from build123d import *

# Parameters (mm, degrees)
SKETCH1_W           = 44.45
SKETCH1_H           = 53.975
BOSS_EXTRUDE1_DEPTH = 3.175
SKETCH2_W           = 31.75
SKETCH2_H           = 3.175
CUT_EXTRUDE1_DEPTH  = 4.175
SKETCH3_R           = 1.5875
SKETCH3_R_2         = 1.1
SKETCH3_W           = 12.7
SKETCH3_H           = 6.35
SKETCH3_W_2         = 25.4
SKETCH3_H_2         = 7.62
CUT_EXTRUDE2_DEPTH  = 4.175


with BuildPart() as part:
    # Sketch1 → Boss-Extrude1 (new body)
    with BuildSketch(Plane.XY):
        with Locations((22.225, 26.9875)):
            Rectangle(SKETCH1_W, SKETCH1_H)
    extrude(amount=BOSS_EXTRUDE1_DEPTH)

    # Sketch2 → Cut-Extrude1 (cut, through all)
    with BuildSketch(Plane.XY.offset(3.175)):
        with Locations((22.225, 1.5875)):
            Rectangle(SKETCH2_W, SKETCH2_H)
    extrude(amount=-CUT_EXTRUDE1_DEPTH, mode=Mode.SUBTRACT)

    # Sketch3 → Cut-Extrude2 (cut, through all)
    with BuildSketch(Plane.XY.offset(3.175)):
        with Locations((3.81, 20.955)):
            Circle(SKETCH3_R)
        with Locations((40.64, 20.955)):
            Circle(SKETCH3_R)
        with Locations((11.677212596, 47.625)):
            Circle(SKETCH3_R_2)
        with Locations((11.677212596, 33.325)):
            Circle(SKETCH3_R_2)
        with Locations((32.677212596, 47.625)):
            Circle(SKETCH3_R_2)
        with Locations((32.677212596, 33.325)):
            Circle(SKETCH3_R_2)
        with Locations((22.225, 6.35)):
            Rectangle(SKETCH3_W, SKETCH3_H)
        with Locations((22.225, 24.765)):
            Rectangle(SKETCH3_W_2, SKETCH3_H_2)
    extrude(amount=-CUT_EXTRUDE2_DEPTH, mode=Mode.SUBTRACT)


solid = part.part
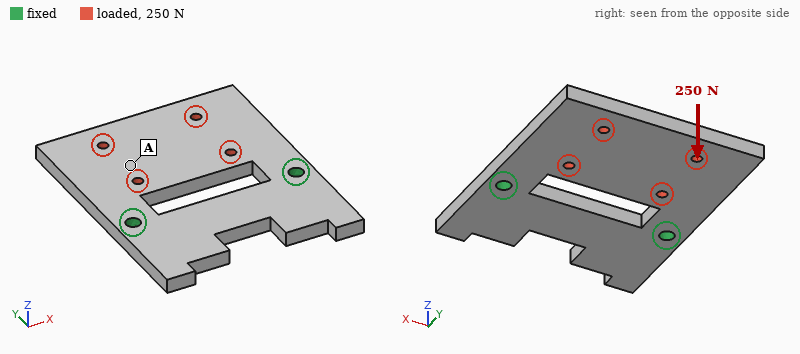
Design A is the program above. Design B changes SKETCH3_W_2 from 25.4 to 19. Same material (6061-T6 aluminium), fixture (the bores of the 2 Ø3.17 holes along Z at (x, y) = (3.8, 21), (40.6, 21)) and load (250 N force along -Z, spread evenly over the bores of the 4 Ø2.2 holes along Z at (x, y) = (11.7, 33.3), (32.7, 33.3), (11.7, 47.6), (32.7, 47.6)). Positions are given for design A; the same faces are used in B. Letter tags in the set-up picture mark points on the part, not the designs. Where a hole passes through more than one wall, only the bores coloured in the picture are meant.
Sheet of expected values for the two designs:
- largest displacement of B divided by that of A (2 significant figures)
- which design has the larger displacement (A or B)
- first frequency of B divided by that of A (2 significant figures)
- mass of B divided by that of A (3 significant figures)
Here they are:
0.83
A
1.1
1.02
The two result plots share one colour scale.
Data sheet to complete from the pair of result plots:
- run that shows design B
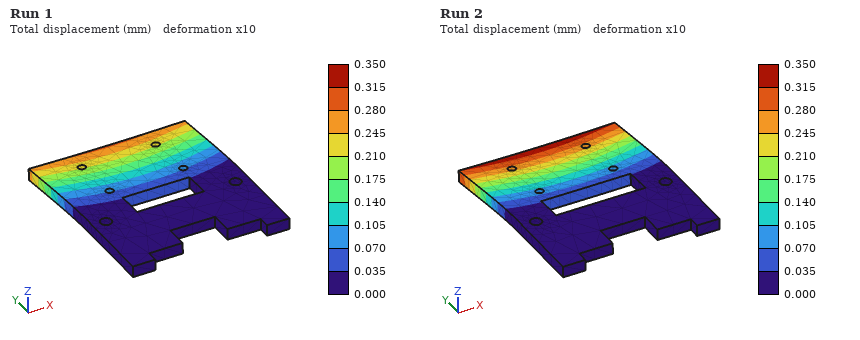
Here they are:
Run 1
